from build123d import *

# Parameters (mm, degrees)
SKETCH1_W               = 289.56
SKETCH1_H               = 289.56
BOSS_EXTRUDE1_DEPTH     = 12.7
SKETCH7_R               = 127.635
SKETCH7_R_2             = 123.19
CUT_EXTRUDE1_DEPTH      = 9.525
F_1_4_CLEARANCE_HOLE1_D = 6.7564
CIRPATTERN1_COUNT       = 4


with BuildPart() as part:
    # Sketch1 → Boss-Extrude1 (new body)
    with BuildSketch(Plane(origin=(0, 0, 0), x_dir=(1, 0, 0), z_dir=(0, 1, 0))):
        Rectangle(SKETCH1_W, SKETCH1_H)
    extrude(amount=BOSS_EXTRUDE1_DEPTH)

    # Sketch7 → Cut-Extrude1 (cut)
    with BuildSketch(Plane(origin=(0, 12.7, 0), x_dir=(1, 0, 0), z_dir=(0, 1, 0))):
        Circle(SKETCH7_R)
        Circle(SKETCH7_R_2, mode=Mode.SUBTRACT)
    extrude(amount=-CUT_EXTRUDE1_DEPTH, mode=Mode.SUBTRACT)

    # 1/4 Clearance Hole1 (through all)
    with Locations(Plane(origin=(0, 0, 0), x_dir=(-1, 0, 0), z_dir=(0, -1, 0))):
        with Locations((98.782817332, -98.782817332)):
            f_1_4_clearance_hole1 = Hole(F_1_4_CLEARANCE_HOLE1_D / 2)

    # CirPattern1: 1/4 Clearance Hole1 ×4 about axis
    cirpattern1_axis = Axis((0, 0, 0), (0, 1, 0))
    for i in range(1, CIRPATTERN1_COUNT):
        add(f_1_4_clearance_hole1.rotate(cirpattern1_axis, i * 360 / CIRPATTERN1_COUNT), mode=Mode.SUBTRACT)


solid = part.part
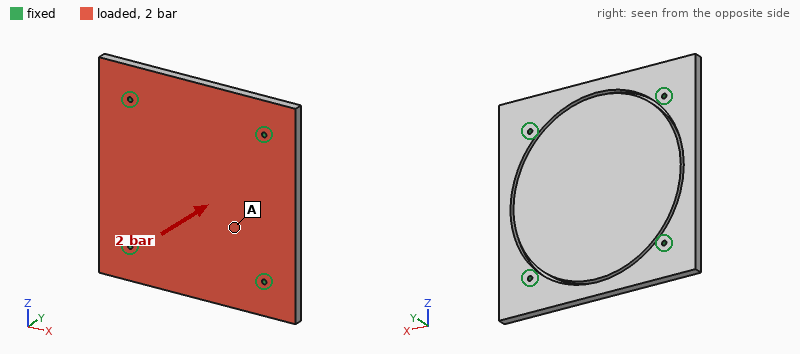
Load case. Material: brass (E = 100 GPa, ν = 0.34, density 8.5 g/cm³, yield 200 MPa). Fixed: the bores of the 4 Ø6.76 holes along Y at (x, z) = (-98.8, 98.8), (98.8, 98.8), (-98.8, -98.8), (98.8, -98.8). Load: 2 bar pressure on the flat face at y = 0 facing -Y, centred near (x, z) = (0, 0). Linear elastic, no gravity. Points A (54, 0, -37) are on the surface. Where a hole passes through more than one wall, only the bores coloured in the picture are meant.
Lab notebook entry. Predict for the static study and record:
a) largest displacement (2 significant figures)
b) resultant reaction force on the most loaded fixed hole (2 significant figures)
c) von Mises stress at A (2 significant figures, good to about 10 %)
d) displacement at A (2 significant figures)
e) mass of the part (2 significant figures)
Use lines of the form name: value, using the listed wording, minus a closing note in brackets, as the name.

largest displacement: 0.17 mm
resultant reaction force on the most loaded fixed hole: 5.2 kN
von Mises stress at A: 13 MPa
displacement at A: 0.13 mm
mass of the part: 8.8 kg
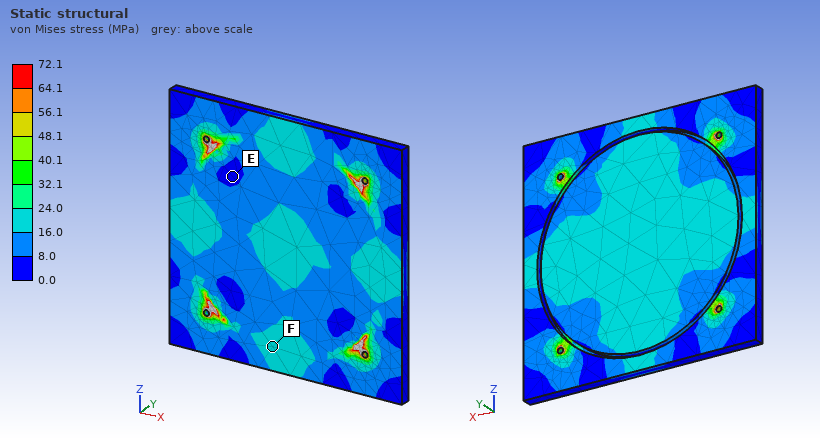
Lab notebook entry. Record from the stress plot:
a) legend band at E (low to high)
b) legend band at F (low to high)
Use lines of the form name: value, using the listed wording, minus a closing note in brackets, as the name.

legend band at E: 0.0 to 8.0 MPa
legend band at F: 16.0 to 24.0 MPa
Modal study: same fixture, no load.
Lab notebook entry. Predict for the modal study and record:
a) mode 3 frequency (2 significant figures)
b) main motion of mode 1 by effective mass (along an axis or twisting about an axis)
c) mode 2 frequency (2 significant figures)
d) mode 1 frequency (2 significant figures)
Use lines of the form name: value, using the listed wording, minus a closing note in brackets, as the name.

mode 3 frequency: 960 Hz
main motion of mode 1 by effective mass: along Y
mode 2 frequency: 910 Hz
mode 1 frequency: 630 Hz
